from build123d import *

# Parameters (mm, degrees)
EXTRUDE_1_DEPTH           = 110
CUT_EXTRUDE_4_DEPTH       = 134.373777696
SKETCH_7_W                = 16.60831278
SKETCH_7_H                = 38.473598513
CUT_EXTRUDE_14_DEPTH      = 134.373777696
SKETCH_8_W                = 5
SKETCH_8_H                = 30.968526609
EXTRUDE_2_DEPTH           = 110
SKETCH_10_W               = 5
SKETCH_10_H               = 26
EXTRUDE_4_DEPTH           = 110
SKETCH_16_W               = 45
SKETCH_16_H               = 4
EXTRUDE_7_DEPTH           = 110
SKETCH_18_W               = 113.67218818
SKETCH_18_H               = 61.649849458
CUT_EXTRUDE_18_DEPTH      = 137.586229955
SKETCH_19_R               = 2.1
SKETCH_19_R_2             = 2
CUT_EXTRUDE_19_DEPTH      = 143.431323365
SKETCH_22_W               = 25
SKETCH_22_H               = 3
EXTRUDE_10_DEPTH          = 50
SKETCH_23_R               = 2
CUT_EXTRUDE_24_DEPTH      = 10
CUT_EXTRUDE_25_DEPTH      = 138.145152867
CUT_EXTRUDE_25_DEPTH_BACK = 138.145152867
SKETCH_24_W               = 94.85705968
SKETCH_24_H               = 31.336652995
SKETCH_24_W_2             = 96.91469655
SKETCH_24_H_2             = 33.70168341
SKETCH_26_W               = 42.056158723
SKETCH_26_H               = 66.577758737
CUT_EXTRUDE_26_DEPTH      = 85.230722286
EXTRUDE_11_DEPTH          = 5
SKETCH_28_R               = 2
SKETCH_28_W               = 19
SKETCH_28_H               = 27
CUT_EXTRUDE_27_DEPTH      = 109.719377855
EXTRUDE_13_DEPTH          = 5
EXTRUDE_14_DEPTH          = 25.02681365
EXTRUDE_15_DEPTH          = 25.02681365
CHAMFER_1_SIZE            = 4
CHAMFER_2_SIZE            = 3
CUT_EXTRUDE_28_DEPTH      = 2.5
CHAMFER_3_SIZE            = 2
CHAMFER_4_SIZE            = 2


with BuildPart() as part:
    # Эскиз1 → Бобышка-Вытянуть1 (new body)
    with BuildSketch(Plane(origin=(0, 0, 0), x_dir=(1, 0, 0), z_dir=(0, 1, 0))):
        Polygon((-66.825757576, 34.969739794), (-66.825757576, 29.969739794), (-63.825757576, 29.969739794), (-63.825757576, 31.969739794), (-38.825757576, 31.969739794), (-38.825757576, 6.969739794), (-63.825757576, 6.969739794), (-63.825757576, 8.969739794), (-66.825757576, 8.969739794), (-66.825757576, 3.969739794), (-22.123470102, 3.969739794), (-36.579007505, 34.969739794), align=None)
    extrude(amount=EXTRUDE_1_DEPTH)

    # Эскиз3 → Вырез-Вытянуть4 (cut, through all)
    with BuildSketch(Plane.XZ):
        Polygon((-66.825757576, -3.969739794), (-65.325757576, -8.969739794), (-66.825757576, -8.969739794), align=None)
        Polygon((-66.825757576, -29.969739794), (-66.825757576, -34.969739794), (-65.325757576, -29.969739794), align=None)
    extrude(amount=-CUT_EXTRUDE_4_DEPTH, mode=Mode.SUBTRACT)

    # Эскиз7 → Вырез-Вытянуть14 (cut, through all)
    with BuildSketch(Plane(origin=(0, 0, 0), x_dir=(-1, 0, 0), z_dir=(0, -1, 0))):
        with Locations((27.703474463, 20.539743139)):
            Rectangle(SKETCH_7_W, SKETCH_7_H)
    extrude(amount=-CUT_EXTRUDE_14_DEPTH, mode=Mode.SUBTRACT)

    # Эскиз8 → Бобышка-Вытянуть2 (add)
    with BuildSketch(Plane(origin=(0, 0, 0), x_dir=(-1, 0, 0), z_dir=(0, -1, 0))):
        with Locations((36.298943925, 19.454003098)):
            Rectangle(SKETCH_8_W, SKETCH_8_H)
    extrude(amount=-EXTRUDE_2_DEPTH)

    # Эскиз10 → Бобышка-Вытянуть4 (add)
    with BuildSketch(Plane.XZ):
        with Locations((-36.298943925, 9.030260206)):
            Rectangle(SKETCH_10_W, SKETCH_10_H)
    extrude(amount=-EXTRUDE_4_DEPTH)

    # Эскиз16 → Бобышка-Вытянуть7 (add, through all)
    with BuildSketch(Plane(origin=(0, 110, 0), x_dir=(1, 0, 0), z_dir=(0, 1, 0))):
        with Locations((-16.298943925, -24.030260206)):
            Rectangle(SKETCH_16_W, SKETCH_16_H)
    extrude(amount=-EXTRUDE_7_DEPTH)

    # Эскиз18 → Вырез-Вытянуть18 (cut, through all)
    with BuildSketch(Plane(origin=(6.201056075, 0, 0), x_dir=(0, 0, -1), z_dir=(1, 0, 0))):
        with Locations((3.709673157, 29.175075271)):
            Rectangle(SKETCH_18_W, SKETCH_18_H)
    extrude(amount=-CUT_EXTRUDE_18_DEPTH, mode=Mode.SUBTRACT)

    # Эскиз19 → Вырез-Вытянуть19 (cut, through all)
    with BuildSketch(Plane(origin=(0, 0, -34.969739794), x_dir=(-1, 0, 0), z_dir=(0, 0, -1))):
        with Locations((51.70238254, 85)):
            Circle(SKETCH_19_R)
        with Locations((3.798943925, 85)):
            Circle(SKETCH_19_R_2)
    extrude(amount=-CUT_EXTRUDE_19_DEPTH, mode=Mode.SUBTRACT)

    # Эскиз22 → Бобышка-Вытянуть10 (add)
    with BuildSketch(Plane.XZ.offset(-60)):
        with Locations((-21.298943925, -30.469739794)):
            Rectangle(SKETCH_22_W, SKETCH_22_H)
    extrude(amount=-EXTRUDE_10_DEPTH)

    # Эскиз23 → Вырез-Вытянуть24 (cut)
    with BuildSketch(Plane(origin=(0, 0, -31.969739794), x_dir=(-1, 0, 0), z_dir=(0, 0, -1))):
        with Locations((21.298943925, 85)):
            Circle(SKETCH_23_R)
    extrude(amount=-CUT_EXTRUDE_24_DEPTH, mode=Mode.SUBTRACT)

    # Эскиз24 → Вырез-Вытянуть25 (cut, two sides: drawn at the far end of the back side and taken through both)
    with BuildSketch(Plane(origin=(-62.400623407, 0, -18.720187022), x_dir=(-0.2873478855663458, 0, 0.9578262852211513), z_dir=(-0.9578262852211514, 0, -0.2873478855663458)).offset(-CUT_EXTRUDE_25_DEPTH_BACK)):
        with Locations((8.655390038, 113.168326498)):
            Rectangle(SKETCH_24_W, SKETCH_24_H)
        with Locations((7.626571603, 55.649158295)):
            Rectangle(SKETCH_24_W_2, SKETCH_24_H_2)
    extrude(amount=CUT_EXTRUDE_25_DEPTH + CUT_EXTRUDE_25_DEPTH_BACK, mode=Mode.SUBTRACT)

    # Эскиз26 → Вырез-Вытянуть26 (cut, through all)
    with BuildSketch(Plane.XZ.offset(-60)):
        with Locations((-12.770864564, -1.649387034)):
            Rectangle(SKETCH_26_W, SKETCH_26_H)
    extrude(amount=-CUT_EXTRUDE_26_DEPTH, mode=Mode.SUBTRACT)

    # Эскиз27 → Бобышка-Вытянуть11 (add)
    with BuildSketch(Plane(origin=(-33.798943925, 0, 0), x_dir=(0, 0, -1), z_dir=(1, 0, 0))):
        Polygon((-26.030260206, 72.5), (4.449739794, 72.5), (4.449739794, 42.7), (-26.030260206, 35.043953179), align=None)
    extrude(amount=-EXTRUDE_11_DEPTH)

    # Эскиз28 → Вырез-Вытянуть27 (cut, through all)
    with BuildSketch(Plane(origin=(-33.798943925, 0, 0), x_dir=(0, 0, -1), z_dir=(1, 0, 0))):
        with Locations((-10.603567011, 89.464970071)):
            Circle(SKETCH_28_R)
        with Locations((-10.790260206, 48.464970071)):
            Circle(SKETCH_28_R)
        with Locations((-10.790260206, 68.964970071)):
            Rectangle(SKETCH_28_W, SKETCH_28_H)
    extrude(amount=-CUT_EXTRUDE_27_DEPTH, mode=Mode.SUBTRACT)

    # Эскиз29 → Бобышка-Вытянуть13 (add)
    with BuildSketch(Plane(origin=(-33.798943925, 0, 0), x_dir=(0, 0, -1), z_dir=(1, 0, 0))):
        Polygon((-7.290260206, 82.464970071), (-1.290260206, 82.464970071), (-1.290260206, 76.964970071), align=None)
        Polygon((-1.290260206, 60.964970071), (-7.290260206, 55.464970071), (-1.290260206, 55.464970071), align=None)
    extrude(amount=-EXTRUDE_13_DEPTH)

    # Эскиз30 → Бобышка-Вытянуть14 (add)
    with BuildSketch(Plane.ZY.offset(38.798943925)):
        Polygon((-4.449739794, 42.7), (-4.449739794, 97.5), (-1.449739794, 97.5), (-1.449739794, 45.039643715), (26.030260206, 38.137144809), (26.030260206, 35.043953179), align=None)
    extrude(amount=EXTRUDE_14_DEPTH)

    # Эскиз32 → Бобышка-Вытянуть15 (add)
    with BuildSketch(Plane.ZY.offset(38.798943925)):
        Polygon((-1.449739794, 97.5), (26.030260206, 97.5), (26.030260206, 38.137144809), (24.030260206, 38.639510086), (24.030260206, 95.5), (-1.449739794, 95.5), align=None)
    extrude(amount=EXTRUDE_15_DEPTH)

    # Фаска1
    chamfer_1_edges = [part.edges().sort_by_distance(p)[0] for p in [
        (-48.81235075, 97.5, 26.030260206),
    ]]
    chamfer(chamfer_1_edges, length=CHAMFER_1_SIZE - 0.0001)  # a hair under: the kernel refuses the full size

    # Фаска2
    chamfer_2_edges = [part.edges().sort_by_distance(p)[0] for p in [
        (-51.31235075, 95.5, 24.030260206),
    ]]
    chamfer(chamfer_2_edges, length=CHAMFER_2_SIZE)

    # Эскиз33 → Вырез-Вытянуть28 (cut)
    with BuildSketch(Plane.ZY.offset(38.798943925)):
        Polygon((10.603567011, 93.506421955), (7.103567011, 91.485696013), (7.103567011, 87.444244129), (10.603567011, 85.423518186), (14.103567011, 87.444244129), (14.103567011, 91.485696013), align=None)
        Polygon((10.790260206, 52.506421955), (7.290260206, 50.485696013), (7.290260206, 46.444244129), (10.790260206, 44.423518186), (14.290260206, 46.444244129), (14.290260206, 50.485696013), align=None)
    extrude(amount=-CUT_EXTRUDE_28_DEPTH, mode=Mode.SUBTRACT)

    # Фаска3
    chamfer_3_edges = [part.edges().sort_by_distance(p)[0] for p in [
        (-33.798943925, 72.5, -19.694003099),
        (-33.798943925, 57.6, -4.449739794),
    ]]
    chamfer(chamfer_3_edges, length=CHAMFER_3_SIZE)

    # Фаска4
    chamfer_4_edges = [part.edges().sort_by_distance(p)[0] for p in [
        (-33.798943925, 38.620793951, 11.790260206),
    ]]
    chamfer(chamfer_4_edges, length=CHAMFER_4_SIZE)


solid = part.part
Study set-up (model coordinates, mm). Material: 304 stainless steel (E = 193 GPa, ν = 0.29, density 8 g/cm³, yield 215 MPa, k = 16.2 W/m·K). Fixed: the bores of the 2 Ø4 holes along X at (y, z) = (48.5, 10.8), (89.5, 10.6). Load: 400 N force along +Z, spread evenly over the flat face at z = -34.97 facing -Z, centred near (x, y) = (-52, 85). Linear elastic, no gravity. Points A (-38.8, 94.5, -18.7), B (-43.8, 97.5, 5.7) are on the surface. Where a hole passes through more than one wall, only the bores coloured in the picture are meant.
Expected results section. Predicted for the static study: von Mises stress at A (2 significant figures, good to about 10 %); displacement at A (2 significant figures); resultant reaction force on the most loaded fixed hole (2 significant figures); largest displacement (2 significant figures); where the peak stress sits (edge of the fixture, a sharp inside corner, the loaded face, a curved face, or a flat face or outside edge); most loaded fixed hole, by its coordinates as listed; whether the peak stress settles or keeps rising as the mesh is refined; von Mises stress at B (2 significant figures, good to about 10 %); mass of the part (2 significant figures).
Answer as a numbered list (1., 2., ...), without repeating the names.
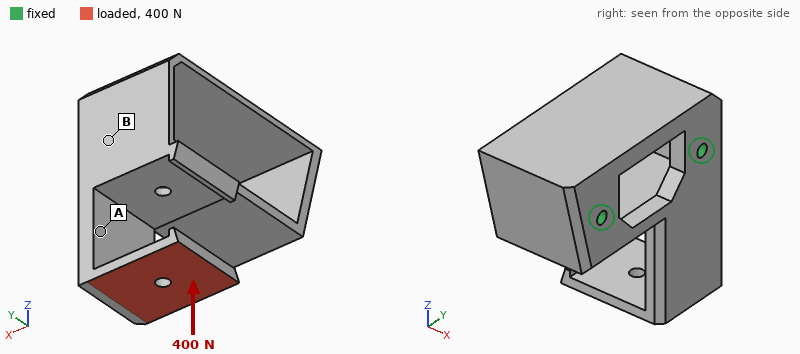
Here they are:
1. 63 MPa
2. 0.049 mm
3. 350 N
4. 0.28 mm
5. edge of the fixture
6. (89.5, 10.6)
7. keeps rising
8. 15 MPa
9. 190 g
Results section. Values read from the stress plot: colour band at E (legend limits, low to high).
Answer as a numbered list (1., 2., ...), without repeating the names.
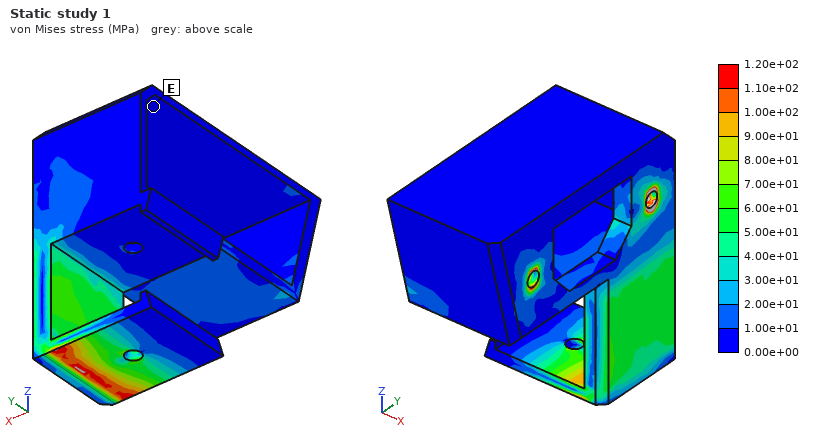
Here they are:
1. 0.00e+00 to 1.00e+01 MPa
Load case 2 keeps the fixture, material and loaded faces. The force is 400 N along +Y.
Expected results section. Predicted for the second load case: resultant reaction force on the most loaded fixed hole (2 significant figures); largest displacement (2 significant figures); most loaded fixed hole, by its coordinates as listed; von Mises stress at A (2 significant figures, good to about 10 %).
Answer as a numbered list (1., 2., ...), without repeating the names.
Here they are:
1. 600 N
2. 94 µm
3. (48.5, 10.8)
4. 49 MPa
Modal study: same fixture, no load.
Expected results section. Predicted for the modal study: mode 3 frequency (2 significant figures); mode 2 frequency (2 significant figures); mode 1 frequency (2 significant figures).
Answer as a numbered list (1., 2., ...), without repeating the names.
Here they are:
1. 2600 Hz
2. 2200 Hz
3. 1000 Hz
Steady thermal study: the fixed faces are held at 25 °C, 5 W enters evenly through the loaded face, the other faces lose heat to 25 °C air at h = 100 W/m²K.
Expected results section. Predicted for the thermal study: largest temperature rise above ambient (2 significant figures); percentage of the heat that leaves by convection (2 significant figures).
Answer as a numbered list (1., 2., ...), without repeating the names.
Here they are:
1. 33 K
2. 97 %
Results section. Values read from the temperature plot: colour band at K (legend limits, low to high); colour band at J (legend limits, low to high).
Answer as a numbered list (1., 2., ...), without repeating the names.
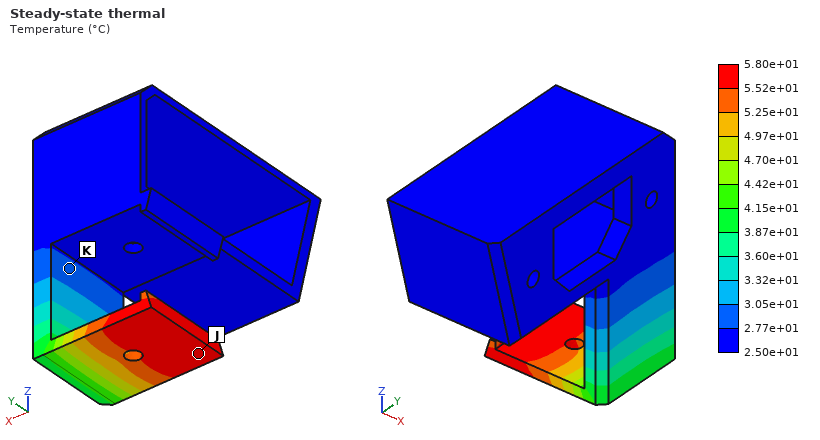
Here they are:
1. 2.77e+01 to 3.05e+01 °C
2. 5.52e+01 to 5.80e+01 °C
